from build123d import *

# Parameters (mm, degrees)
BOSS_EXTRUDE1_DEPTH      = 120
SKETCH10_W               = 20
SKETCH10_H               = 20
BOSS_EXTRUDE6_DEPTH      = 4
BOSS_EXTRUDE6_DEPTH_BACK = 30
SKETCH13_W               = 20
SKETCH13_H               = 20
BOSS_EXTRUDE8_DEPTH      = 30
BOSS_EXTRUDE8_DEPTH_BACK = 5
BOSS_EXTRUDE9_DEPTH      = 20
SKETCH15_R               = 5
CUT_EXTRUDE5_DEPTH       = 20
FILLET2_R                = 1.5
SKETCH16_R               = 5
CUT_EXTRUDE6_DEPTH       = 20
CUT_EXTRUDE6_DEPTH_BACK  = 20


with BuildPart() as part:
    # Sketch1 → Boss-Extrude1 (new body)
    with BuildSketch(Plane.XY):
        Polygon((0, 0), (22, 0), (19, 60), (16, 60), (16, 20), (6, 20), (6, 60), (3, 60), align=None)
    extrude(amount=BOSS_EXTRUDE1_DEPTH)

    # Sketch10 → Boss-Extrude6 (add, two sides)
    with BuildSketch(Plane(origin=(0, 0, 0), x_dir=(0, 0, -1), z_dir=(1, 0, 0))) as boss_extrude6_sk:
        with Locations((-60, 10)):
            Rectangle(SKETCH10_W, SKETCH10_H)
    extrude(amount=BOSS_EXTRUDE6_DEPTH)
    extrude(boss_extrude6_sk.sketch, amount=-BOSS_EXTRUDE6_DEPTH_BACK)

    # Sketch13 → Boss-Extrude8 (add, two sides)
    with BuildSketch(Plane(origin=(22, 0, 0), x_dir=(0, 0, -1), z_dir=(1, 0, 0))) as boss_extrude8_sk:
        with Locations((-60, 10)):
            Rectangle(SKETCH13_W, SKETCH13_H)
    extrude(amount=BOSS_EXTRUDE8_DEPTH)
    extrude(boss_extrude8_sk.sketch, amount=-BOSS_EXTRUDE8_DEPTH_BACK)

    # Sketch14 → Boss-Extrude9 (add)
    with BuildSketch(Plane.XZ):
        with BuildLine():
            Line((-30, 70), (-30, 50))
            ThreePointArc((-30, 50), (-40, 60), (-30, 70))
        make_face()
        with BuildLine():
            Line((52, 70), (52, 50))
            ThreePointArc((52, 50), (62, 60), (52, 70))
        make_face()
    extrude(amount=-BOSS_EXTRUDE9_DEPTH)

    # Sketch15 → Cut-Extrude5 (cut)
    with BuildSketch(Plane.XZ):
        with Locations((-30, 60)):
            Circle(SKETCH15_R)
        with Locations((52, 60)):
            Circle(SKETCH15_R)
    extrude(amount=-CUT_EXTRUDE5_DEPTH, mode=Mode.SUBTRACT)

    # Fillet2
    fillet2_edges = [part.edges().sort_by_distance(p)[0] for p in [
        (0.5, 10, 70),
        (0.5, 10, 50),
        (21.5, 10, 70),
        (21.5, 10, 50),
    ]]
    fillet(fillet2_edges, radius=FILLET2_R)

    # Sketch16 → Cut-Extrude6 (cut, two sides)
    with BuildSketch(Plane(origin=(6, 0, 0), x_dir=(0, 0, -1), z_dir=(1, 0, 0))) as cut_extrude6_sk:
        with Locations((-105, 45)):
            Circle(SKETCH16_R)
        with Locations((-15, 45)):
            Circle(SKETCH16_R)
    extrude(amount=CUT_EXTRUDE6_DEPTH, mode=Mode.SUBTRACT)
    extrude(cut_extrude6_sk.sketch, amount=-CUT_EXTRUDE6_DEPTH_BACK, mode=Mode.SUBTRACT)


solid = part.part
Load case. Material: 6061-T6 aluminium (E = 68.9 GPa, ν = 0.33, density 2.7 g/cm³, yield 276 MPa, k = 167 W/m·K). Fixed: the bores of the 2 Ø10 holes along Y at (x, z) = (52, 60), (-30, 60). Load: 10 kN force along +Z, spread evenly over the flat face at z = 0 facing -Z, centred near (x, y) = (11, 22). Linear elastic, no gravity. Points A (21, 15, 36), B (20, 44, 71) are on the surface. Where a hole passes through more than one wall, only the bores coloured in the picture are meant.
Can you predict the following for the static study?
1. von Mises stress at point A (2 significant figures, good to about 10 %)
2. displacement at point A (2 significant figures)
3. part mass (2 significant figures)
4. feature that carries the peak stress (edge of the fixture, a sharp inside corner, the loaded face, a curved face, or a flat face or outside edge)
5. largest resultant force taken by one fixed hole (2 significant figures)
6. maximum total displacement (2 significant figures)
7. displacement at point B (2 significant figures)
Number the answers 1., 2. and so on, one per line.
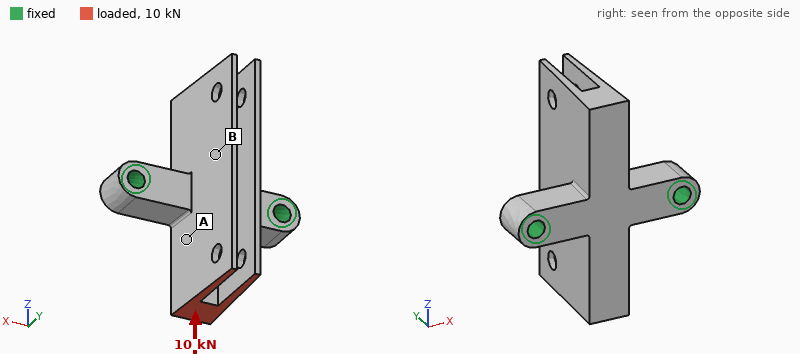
1. 17 MPa
2. 0.098 mm
3. 310 g
4. a curved face
5. 5.0 kN
6. 0.30 mm
7. 0.16 mm
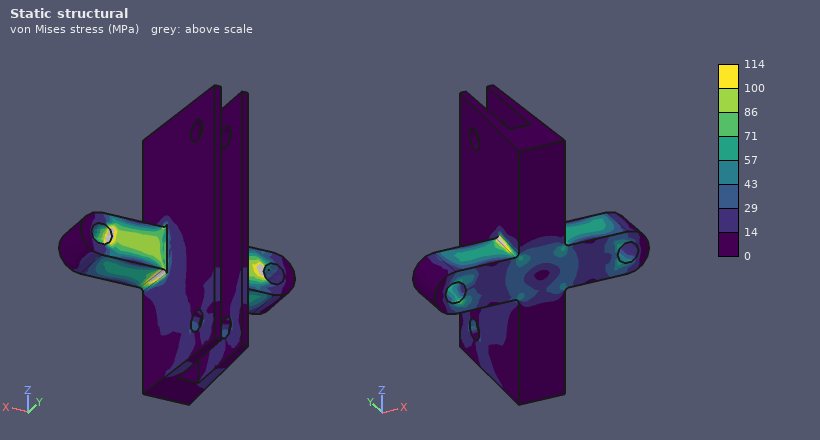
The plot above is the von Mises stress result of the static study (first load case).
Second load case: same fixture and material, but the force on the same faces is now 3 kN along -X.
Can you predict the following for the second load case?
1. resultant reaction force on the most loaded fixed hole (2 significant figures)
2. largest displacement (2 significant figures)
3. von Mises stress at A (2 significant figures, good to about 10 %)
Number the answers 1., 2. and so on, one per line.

1. 3.4 kN
2. 0.63 mm
3. 59 MPa
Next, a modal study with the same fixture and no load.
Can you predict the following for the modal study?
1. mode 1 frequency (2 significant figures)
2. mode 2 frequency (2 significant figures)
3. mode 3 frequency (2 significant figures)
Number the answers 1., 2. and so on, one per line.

1. 1500 Hz
2. 2300 Hz
3. 2400 Hz
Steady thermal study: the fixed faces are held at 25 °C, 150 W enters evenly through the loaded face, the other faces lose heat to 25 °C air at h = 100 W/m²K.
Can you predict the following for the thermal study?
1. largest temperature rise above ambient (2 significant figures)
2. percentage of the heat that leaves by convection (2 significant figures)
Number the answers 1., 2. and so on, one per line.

1. 72 K
2. 53 %
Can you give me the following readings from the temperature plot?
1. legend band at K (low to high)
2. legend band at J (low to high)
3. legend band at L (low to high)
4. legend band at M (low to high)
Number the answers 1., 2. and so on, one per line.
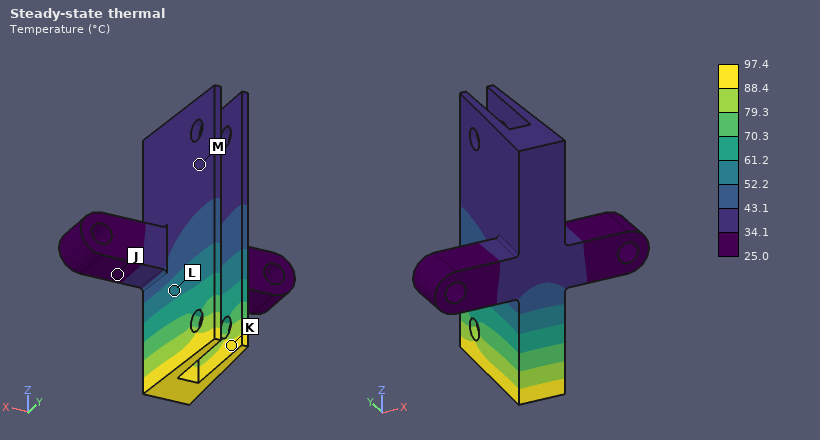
1. 88.4 to 97.4 °C
2. 25.0 to 34.1 °C
3. 52.2 to 61.2 °C
4. 34.1 to 43.1 °C
